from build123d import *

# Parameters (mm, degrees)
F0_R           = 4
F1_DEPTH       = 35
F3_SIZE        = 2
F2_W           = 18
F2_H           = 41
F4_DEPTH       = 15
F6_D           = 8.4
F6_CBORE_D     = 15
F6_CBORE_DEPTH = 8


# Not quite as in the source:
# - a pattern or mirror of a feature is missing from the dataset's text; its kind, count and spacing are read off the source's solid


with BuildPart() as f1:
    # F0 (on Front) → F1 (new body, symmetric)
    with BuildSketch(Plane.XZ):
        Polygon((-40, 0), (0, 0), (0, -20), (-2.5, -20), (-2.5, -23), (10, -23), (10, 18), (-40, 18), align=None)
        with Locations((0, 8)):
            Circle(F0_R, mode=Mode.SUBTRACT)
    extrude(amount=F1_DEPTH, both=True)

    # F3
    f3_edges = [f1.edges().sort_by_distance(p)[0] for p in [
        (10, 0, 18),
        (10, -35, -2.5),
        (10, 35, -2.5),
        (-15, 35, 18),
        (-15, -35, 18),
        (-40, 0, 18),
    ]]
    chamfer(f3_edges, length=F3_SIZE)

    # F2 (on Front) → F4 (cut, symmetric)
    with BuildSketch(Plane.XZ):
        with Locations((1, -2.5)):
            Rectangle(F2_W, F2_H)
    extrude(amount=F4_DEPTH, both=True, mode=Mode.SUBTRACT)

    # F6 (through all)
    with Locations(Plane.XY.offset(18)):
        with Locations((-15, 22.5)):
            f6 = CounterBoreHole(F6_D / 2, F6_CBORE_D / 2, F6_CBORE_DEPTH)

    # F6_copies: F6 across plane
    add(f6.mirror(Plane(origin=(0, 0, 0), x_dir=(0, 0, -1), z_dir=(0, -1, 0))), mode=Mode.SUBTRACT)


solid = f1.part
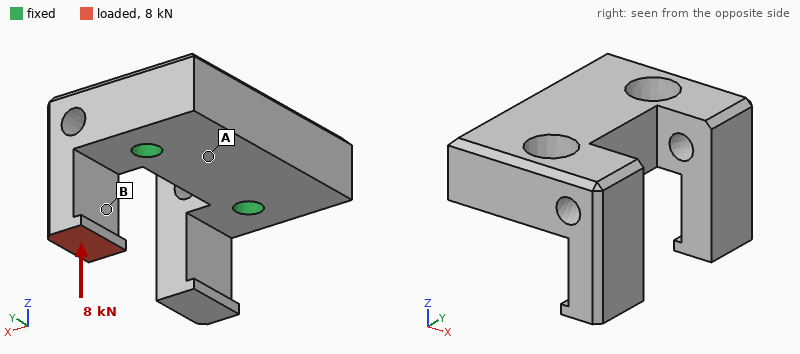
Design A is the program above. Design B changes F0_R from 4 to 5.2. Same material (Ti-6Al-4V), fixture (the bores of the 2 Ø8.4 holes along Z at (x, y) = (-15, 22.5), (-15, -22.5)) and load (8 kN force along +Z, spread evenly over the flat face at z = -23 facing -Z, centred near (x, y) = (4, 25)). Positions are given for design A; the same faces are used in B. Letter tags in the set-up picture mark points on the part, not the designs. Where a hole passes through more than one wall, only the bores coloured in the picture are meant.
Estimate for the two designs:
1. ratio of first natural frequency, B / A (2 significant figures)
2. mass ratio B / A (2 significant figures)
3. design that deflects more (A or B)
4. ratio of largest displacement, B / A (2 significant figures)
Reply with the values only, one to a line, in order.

0.93
0.98
B
1.2
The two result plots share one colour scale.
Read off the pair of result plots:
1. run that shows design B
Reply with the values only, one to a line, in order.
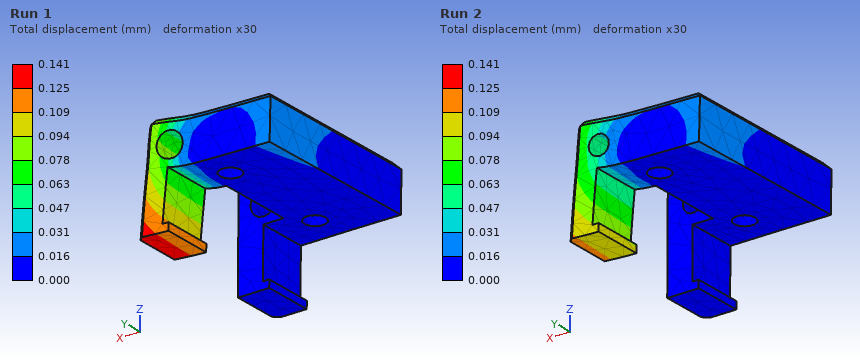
Run 1
